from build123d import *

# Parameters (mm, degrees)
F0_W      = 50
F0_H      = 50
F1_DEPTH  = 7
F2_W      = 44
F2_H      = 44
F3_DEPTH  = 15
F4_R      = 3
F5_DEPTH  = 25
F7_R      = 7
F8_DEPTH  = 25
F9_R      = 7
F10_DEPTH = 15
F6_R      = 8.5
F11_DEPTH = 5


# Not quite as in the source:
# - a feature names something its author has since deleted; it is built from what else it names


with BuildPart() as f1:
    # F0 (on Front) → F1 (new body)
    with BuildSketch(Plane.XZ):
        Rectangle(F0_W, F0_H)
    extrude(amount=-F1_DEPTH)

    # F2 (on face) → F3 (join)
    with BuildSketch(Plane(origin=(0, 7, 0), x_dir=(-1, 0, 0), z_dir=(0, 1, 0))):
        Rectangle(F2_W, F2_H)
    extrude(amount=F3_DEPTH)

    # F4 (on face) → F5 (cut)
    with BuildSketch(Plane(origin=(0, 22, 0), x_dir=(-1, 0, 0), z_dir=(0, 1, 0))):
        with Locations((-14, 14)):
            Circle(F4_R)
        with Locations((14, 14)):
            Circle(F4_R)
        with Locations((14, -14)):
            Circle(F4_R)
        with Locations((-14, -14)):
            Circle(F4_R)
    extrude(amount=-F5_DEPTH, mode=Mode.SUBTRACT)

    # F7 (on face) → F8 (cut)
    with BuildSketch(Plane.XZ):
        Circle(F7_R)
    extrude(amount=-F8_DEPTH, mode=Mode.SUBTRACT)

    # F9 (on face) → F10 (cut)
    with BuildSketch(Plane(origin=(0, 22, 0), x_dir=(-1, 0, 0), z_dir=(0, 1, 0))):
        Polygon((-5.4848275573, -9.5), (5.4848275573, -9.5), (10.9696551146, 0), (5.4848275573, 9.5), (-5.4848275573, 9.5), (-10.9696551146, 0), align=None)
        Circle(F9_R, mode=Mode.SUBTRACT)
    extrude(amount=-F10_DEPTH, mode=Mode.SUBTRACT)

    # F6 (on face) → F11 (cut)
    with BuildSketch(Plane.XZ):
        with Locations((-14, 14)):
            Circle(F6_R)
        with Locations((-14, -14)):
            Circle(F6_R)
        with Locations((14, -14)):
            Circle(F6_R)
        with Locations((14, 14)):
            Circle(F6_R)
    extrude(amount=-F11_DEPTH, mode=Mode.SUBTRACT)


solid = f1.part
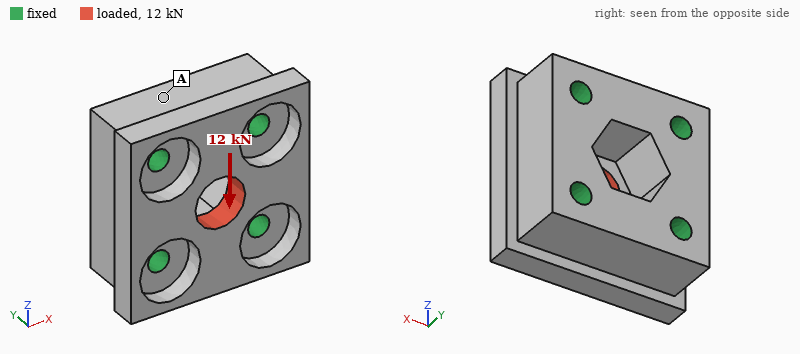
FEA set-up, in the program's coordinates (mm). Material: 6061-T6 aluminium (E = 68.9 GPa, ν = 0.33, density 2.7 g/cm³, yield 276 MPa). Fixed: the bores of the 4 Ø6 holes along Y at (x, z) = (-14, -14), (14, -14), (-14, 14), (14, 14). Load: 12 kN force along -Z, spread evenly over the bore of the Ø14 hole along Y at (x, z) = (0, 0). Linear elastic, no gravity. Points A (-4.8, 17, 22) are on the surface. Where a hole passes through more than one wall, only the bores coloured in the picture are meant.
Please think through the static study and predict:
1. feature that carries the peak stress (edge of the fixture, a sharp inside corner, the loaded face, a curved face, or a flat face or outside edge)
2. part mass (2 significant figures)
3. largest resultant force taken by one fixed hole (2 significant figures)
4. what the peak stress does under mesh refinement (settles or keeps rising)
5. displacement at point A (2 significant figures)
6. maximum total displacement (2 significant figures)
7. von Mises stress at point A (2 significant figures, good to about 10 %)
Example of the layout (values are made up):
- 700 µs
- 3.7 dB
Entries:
- edge of the fixture
- 93 g
- 3.3 kN
- keeps rising
- 2.4 µm
- 16 µm
- 11 MPa
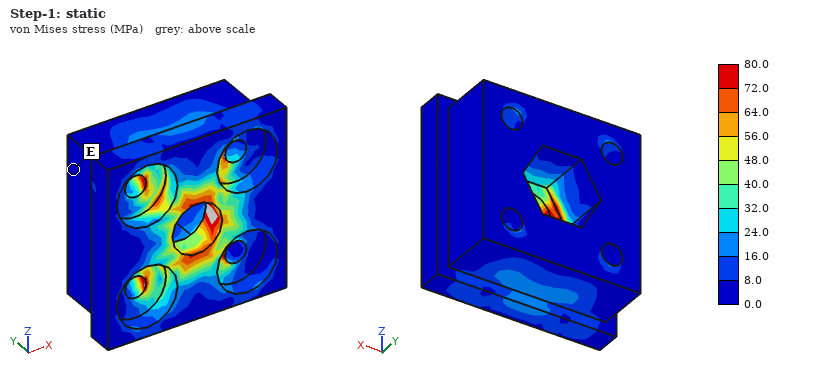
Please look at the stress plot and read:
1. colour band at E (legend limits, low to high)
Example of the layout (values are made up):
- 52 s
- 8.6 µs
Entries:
- 0.0 to 8.0 MPa
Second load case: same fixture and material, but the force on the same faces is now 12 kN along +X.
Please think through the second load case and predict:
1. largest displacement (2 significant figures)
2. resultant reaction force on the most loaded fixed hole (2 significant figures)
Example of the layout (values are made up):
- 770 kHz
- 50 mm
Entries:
- 16 µm
- 3.3 kN
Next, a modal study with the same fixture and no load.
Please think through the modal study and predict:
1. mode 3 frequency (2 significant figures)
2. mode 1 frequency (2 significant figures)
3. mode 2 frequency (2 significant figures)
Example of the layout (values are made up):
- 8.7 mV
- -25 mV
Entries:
- 37 kHz
- 34 kHz
- 37 kHz
